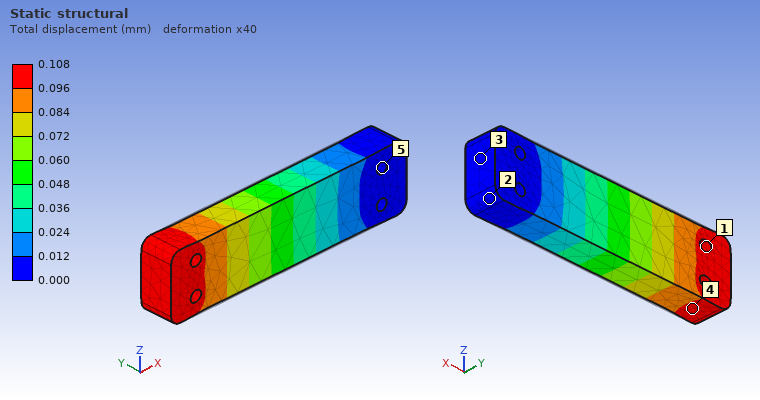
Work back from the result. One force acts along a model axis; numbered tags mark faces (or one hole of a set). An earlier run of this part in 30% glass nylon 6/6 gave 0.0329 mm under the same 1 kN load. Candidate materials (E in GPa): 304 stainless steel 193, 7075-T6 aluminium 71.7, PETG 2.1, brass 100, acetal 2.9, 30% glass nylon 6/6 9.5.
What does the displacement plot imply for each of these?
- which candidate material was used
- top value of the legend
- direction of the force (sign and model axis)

acetal
0.108 mm
-X
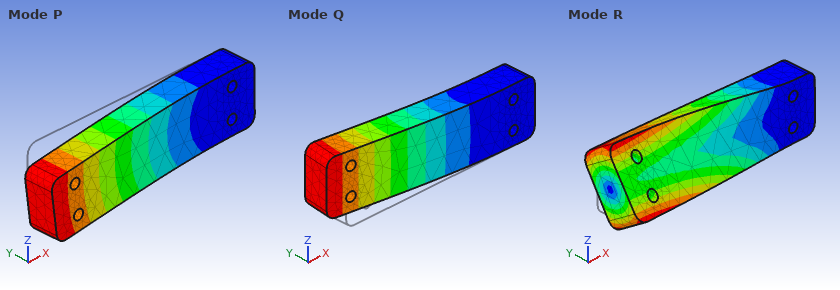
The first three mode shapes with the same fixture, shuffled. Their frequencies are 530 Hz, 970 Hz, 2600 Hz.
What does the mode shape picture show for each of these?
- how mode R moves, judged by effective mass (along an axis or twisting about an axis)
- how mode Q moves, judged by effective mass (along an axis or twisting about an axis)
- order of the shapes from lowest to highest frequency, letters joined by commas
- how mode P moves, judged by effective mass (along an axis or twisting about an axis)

twisting about X
along Y
Q, P, R
along Z
